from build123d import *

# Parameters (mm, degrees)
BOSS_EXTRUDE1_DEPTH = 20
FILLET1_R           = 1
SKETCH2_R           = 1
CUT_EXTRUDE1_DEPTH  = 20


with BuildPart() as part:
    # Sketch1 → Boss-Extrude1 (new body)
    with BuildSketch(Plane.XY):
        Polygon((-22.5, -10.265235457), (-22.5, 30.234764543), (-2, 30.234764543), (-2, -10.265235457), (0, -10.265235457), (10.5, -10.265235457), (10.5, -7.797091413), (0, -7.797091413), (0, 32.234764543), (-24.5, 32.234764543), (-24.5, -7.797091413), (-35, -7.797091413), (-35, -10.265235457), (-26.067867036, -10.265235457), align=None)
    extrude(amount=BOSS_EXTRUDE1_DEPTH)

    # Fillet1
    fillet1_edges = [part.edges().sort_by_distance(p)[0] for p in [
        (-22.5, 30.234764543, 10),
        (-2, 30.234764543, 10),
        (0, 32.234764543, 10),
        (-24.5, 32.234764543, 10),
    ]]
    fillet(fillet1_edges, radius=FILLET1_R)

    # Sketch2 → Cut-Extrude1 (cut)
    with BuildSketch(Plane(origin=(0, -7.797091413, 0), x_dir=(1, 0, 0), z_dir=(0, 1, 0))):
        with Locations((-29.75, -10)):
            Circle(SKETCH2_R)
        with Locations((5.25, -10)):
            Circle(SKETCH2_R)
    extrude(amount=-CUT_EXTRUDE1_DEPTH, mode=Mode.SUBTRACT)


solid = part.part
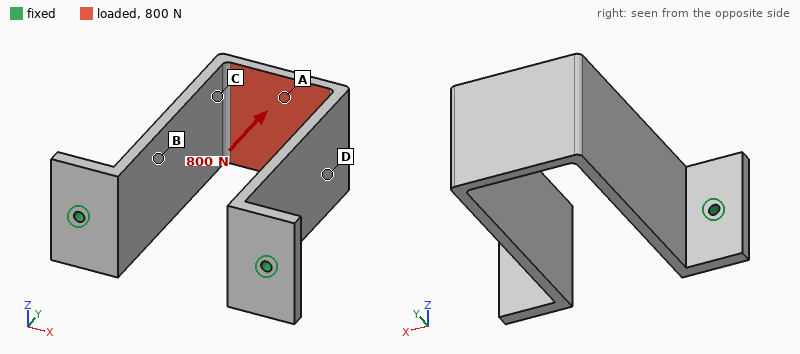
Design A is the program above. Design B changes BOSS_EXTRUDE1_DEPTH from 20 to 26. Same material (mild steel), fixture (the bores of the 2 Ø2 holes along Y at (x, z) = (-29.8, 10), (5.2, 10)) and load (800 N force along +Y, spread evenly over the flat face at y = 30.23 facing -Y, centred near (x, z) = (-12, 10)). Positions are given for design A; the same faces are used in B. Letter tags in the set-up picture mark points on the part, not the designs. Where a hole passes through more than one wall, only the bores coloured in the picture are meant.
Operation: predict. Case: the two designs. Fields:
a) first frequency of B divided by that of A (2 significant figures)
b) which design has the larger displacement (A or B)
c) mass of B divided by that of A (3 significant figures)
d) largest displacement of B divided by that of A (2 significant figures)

0.98
B
1.30
1.8
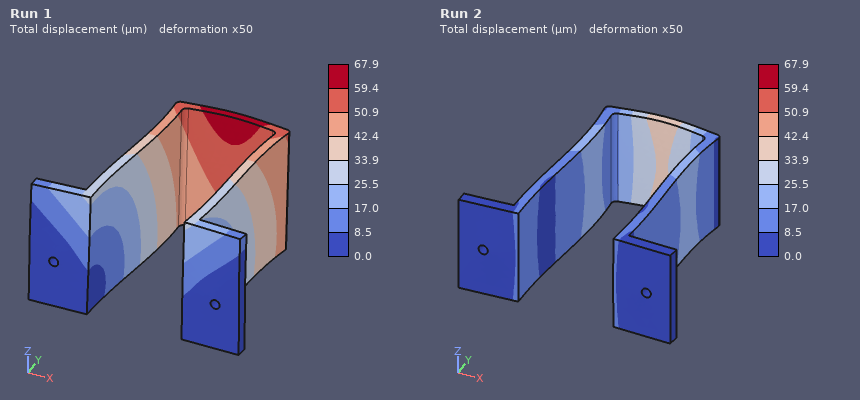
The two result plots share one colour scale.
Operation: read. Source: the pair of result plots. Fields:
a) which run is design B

Run 1
